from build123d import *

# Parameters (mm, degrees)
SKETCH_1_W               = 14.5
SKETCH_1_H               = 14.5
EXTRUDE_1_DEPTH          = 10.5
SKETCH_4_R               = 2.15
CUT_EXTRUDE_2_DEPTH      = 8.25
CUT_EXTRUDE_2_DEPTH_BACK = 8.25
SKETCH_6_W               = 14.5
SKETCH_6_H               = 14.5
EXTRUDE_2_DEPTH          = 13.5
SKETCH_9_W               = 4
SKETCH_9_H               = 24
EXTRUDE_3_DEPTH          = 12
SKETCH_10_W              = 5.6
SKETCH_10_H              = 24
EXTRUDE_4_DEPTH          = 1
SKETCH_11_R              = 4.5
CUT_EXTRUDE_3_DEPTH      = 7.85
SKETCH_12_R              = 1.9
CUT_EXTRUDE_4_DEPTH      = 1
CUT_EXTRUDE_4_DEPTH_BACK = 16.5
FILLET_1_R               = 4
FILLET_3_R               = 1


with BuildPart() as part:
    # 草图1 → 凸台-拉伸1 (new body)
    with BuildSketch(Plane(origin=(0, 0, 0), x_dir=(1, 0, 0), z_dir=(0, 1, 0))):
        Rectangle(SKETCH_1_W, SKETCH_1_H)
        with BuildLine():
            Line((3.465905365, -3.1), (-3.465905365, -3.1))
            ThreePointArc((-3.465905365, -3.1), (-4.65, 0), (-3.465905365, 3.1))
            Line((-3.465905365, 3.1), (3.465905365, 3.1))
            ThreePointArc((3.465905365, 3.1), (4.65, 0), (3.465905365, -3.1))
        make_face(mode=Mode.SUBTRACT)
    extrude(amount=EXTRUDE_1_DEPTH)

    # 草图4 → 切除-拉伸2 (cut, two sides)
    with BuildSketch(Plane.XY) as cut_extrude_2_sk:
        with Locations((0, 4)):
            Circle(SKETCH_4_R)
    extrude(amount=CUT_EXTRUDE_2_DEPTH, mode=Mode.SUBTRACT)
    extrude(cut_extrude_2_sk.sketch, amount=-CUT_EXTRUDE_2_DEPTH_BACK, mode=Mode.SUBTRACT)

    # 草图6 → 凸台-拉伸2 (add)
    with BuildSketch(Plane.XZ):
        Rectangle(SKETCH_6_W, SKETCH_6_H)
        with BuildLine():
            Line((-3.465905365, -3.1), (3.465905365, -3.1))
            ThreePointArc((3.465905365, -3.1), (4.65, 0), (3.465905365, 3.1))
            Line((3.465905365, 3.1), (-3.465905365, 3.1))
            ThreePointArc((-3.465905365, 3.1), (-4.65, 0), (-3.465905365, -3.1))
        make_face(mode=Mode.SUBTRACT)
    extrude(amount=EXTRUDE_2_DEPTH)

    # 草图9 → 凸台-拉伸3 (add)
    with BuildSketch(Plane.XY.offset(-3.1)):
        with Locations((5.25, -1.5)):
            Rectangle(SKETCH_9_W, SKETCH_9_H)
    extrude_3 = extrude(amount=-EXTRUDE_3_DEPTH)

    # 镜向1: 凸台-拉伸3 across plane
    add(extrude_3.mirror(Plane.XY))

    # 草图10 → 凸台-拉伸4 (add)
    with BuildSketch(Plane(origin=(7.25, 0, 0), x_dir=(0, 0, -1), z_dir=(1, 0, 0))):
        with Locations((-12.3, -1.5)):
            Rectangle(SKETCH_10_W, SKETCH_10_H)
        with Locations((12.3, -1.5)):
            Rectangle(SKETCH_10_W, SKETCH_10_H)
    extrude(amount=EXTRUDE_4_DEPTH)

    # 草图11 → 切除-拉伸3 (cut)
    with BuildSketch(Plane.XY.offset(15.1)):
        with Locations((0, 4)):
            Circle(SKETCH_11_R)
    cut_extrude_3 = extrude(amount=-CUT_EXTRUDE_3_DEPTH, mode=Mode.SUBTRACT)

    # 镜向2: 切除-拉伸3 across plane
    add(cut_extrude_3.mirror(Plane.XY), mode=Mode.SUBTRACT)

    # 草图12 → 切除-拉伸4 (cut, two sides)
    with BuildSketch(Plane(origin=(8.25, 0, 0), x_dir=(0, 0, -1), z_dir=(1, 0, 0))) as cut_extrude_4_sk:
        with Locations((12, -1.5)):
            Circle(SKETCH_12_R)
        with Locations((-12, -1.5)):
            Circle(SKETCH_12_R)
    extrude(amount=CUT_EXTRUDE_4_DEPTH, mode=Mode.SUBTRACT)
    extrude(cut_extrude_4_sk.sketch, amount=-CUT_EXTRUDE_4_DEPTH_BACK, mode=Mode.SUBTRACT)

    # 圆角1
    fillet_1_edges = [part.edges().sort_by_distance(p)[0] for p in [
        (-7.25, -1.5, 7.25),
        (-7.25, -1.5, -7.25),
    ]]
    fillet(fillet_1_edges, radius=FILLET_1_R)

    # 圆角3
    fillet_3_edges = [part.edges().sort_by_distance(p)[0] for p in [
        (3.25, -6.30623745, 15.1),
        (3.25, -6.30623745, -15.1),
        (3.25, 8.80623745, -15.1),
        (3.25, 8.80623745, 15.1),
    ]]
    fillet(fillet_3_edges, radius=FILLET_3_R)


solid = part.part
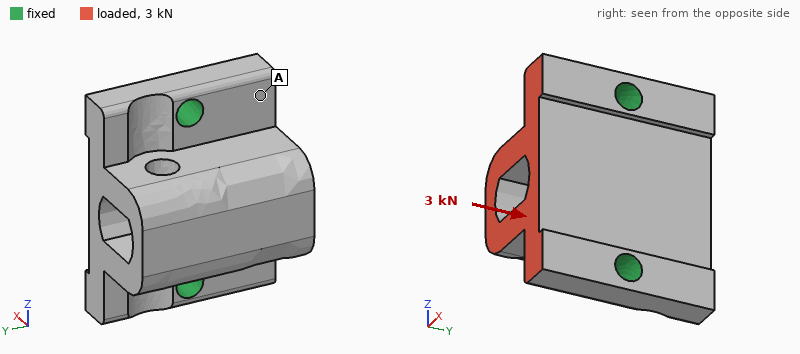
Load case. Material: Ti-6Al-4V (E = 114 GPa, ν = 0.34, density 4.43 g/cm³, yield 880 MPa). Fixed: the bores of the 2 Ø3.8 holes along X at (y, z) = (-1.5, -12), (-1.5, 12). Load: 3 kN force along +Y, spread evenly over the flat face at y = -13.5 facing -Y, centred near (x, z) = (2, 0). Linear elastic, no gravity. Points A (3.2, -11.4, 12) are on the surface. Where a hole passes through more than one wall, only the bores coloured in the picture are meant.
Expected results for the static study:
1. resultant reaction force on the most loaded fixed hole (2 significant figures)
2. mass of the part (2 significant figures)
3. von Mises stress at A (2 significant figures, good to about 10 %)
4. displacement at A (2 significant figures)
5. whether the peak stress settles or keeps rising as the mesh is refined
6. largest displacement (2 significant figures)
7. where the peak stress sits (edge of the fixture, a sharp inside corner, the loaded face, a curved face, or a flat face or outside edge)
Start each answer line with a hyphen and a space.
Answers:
- 1.5 kN
- 22 g
- 23 MPa
- 9.8 µm
- keeps rising
- 28 µm
- edge of the fixture
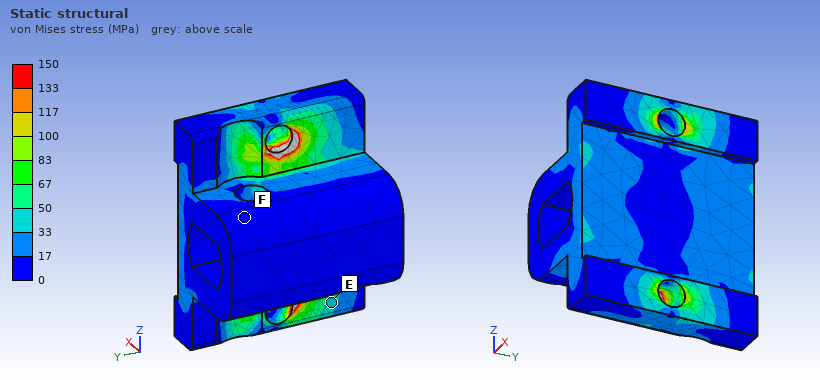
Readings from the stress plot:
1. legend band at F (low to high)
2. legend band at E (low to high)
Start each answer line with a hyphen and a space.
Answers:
- 0 to 17 MPa
- 33 to 50 MPa
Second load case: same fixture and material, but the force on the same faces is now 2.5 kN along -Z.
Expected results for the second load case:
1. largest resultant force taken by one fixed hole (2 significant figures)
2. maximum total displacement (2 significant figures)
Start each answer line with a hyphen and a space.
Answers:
- 1.7 kN
- 16 µm
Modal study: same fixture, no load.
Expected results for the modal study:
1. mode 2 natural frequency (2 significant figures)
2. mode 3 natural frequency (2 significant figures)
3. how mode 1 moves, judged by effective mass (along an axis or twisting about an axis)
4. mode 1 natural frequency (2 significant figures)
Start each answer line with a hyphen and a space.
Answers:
- 22 kHz
- 22 kHz
- along Y
- 11 kHz
